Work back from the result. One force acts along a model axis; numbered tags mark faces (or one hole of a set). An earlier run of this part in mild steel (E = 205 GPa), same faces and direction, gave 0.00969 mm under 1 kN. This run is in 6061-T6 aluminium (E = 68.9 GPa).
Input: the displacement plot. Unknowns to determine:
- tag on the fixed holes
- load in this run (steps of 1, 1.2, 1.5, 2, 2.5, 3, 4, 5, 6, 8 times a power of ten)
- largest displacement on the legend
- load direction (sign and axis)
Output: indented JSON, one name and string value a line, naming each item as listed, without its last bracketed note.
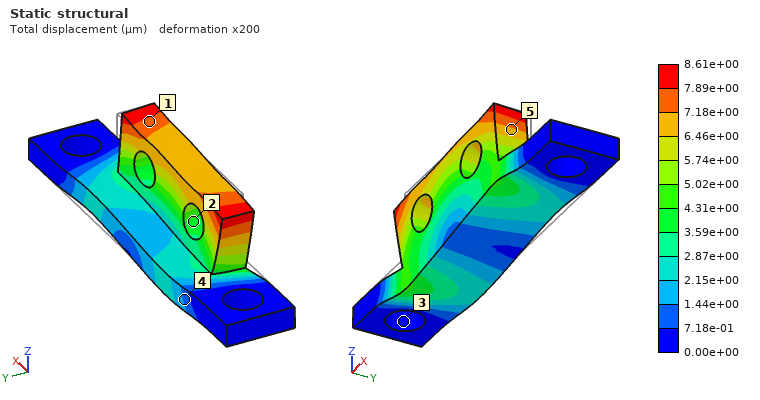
{
  "tag on the fixed holes": "3",
  "load in this run": "300 N",
  "largest displacement on the legend": "8.61e+00 µm",
  "load direction": "-X"
}
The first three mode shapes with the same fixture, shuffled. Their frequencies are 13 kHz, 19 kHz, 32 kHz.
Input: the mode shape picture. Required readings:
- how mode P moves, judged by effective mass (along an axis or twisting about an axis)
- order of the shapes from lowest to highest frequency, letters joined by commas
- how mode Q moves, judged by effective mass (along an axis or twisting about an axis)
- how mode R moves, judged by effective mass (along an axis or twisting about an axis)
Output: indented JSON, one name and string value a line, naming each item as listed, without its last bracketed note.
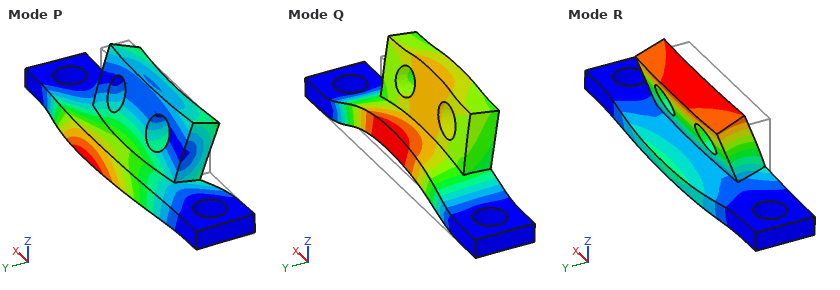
{
  "how mode P moves, judged by effective mass": "along Y",
  "order of the shapes from lowest to highest frequency, letters joined by commas": "R, Q, P",
  "how mode Q moves, judged by effective mass": "along Z",
  "how mode R moves, judged by effective mass": "along Y"
}
